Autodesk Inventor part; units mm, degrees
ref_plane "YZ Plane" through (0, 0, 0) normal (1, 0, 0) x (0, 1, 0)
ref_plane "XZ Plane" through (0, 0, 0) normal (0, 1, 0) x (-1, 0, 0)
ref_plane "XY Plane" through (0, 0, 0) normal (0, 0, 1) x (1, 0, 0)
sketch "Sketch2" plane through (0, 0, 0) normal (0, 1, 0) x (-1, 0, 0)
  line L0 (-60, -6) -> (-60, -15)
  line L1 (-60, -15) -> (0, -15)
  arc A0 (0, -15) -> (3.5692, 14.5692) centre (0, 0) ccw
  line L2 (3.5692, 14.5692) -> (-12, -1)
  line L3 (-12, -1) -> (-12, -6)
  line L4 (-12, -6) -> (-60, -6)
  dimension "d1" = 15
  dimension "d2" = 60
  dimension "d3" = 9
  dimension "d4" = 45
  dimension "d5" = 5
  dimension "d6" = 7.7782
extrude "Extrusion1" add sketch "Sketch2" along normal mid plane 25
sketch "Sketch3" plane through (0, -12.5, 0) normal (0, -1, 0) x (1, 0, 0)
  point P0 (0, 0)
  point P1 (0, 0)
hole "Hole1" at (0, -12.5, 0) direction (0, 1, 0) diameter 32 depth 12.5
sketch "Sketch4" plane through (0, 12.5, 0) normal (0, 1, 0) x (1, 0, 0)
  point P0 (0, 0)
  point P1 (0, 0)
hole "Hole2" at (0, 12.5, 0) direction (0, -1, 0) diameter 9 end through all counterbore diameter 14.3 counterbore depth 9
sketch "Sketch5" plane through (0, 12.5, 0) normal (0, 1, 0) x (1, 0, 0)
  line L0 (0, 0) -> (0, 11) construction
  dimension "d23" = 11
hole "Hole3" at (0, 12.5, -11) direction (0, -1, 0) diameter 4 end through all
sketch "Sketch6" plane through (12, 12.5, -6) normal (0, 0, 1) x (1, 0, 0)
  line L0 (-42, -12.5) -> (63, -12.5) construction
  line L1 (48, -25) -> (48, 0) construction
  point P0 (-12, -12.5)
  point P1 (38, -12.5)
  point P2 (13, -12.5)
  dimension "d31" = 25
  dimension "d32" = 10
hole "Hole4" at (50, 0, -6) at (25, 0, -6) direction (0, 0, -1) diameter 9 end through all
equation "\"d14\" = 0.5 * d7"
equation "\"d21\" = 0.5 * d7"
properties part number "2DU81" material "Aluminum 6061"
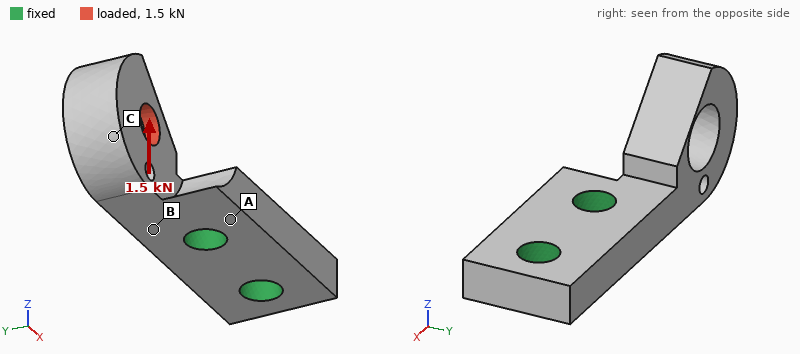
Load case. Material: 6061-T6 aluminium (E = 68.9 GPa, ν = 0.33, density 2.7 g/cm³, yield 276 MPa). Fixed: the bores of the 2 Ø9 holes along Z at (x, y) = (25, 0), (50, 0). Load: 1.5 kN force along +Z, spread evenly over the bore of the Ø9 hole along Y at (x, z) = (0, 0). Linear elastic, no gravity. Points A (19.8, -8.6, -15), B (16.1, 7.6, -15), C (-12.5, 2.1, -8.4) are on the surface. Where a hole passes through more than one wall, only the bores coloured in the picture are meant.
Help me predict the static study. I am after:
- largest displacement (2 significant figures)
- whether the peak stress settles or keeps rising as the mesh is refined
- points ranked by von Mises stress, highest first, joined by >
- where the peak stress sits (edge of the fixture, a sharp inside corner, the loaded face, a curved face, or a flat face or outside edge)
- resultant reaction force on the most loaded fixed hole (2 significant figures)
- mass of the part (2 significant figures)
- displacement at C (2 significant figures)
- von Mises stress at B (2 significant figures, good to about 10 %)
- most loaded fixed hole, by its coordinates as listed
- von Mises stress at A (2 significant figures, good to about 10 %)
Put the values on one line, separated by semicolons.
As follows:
0.21 mm; keeps rising; B > A > C; edge of the fixture; 1.7 kN; 41 g; 0.18 mm; 98 MPa; (25, 0); 34 MPa
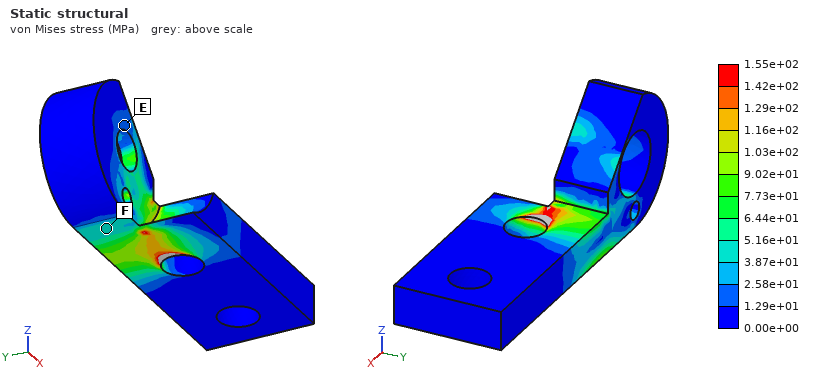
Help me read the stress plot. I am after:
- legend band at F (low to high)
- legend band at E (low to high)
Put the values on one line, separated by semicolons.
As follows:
3.87e+01 to 5.16e+01 MPa; 1.29e+01 to 2.58e+01 MPa
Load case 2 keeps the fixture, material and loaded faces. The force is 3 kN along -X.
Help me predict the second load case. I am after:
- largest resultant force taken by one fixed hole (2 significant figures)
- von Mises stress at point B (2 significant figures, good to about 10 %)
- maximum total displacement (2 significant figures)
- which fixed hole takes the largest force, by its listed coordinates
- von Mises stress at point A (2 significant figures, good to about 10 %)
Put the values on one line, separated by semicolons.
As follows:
2.8 kN; 130 MPa; 0.30 mm; (25, 0); 28 MPa
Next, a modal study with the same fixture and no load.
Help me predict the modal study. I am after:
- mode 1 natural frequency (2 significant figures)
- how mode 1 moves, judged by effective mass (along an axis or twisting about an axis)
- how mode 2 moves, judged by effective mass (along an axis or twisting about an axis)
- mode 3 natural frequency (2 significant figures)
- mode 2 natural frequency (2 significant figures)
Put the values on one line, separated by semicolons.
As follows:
3500 Hz; along Z; along Y; 11 kHz; 4500 Hz
